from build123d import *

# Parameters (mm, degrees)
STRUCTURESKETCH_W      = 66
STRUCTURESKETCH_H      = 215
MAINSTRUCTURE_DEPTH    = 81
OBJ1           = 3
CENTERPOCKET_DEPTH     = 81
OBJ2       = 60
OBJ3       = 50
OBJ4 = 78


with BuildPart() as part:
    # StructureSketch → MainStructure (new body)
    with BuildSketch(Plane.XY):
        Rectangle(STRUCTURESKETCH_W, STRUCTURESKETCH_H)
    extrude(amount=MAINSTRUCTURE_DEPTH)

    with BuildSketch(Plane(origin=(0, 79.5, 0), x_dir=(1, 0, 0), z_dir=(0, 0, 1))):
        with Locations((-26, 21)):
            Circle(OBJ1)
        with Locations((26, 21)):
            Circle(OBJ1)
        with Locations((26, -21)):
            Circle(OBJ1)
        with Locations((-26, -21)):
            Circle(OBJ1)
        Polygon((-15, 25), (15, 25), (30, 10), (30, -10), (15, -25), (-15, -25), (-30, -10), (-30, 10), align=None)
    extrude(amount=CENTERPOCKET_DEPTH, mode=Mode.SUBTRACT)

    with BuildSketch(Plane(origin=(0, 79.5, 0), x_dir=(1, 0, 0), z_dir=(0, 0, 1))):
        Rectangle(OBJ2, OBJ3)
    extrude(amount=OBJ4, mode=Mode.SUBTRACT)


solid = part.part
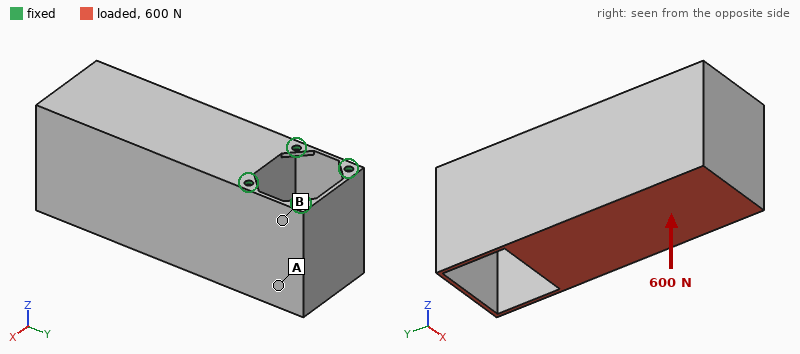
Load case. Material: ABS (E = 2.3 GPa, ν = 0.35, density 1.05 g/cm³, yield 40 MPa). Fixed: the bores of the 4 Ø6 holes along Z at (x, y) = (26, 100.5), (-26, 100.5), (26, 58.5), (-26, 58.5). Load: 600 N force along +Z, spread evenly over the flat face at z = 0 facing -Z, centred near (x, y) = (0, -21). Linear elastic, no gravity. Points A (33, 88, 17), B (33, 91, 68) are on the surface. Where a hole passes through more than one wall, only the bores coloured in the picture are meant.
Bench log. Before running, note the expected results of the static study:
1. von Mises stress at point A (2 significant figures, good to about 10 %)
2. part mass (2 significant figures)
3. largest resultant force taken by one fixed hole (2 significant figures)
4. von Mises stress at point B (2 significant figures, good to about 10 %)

2.6 MPa
950 g
810 N
6.1 MPa
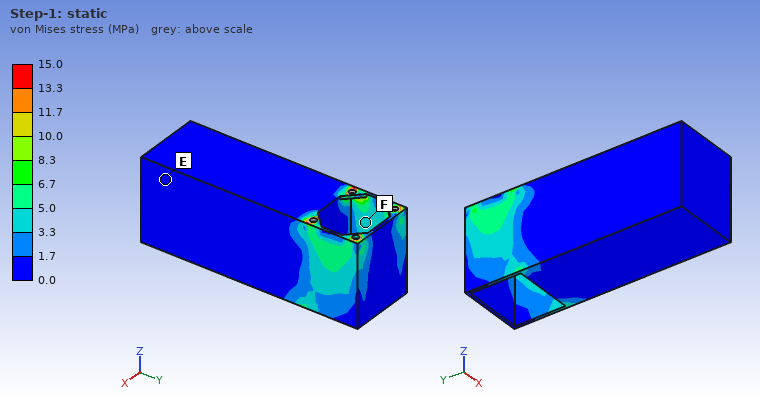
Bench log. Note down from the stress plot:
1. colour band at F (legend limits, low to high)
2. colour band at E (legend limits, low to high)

3.3 to 5.0 MPa
0.0 to 1.7 MPa
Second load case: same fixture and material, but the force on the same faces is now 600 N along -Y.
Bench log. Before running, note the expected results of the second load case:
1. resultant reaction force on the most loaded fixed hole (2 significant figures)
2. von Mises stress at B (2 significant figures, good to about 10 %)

540 N
6.4 MPa
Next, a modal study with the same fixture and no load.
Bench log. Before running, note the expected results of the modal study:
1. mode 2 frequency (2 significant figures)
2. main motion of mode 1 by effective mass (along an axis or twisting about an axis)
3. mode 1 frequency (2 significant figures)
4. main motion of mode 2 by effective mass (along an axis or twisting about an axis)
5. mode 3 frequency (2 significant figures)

210 Hz
along Z
110 Hz
along X
410 Hz
